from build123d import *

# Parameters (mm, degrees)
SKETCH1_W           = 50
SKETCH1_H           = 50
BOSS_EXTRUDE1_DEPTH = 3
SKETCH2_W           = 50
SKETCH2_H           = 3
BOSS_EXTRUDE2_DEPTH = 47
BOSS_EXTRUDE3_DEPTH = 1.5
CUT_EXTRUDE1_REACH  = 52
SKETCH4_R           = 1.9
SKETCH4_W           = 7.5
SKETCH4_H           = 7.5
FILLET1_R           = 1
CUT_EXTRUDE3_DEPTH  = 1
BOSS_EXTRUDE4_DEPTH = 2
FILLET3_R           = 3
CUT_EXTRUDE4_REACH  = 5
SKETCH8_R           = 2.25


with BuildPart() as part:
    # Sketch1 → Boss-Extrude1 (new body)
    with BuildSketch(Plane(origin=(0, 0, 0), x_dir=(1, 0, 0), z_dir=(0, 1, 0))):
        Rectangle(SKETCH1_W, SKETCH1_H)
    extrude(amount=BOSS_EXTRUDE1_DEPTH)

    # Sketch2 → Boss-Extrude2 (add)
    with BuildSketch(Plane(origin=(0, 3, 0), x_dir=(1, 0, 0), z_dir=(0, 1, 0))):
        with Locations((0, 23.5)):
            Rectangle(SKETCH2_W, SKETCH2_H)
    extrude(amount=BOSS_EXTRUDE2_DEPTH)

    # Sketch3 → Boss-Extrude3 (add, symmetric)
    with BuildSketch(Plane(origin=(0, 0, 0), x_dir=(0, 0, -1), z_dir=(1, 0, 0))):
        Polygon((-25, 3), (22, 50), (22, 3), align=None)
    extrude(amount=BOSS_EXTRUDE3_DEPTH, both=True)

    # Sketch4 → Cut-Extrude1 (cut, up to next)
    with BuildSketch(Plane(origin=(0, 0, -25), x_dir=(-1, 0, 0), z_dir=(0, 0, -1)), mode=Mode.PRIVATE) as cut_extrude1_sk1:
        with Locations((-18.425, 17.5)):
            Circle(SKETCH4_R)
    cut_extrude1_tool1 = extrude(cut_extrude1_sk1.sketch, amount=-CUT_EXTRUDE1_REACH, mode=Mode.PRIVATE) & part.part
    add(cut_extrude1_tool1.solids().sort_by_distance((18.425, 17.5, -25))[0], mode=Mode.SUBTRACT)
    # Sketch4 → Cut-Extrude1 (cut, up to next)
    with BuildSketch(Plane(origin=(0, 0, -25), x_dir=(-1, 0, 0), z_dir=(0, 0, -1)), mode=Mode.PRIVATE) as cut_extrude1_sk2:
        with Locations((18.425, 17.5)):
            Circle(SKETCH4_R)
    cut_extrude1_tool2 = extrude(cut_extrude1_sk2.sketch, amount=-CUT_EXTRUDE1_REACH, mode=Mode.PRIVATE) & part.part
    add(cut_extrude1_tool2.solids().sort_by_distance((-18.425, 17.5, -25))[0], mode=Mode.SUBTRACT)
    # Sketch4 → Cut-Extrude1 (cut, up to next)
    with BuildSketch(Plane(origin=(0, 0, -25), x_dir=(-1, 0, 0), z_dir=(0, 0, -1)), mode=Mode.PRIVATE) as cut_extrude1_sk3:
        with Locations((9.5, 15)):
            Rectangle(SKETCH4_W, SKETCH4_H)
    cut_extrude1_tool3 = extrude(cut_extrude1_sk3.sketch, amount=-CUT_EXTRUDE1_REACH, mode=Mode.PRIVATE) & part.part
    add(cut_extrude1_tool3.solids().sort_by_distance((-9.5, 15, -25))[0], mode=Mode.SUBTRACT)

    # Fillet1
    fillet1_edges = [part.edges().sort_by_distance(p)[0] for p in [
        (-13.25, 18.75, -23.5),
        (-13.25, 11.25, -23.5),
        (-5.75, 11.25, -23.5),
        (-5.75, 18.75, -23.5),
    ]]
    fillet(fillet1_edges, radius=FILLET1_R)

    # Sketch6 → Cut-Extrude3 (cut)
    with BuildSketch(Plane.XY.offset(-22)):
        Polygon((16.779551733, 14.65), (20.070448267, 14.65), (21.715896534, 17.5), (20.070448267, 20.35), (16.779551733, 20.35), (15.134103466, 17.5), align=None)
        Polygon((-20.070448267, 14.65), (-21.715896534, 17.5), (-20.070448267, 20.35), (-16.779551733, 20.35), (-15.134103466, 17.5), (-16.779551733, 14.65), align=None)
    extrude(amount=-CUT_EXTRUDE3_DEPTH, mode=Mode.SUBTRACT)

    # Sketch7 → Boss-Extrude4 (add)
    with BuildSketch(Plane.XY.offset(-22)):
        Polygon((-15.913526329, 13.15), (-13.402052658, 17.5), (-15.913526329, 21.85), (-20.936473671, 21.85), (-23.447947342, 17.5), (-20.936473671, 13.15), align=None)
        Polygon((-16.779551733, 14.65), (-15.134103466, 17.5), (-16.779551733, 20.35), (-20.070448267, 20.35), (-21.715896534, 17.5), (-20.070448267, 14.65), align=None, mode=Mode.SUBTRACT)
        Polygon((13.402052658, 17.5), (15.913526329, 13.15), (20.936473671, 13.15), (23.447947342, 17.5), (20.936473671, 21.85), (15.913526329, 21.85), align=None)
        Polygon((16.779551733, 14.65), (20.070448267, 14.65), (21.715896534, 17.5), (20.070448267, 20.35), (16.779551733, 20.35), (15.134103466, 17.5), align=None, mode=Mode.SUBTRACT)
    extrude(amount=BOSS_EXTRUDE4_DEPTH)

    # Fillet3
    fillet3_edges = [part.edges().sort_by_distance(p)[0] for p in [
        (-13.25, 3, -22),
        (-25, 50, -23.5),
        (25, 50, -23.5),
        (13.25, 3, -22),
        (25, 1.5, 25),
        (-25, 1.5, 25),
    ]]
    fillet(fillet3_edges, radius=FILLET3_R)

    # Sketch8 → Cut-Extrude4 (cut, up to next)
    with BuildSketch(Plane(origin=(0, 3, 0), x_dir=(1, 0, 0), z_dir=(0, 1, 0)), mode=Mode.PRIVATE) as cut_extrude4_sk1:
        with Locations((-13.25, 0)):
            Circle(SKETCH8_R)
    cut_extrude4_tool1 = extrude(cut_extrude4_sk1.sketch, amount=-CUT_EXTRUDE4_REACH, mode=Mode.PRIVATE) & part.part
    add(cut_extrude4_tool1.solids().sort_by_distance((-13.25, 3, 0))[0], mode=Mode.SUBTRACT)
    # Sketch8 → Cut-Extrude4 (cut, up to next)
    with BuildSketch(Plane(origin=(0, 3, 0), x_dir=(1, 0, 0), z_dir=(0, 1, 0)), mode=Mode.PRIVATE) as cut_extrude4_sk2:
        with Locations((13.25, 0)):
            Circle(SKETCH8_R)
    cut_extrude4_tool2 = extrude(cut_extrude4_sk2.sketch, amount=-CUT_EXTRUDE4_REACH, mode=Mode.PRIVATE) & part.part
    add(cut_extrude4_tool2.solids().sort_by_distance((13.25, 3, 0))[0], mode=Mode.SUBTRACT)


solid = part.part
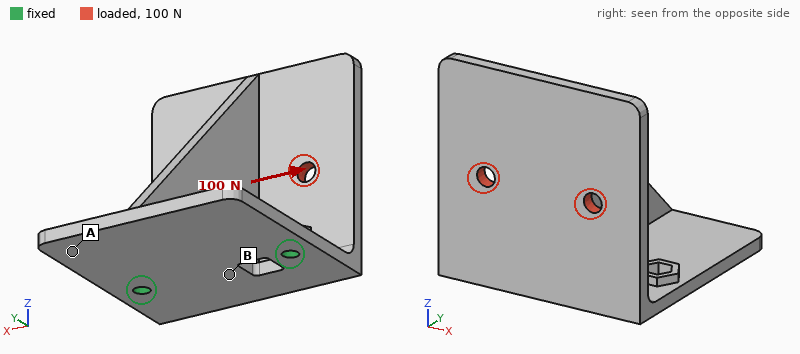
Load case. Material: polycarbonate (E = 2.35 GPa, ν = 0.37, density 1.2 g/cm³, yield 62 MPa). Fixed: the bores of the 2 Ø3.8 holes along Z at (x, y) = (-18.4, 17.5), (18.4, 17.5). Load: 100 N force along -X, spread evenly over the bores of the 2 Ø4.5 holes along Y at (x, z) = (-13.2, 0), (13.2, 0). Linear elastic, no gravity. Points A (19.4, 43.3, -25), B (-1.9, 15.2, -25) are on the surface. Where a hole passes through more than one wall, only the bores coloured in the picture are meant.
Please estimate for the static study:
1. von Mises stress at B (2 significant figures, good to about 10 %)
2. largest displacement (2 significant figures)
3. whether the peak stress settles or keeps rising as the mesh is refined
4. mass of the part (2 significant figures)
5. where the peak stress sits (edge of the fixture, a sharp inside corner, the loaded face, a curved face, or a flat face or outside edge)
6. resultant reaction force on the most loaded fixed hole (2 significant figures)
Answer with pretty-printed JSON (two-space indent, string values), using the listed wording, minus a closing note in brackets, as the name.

{
  "von Mises stress at B": "2.9 MPa",
  "largest displacement": "0.95 mm",
  "whether the peak stress settles or keeps rising as the mesh is refined": "keeps rising",
  "mass of the part": "21 g",
  "where the peak stress sits": "edge of the fixture",
  "resultant reaction force on the most loaded fixed hole": "97 N"
}
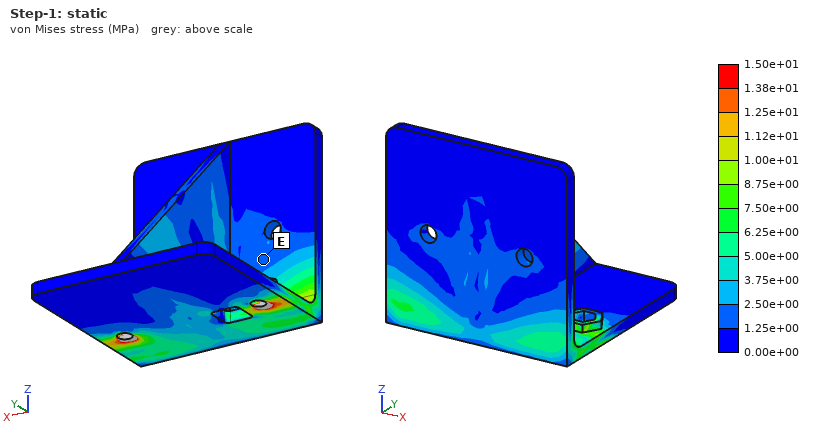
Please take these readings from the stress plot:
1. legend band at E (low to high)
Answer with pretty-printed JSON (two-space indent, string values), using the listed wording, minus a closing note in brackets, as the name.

{
  "legend band at E": "1.25e+00 to 2.50e+00 MPa"
}
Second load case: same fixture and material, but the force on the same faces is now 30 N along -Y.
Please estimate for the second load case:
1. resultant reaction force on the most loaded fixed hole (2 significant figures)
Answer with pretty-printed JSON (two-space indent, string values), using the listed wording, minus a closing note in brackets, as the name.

{
  "resultant reaction force on the most loaded fixed hole": "15 N"
}
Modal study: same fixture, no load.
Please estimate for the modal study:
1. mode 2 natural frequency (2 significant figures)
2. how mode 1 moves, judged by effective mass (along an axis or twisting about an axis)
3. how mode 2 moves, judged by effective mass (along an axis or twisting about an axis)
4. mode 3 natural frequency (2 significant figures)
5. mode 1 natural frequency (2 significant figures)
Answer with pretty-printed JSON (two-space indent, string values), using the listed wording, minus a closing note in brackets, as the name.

{
  "mode 2 natural frequency": "550 Hz",
  "how mode 1 moves, judged by effective mass": "along Y",
  "how mode 2 moves, judged by effective mass": "along X",
  "mode 3 natural frequency": "800 Hz",
  "mode 1 natural frequency": "270 Hz"
}
